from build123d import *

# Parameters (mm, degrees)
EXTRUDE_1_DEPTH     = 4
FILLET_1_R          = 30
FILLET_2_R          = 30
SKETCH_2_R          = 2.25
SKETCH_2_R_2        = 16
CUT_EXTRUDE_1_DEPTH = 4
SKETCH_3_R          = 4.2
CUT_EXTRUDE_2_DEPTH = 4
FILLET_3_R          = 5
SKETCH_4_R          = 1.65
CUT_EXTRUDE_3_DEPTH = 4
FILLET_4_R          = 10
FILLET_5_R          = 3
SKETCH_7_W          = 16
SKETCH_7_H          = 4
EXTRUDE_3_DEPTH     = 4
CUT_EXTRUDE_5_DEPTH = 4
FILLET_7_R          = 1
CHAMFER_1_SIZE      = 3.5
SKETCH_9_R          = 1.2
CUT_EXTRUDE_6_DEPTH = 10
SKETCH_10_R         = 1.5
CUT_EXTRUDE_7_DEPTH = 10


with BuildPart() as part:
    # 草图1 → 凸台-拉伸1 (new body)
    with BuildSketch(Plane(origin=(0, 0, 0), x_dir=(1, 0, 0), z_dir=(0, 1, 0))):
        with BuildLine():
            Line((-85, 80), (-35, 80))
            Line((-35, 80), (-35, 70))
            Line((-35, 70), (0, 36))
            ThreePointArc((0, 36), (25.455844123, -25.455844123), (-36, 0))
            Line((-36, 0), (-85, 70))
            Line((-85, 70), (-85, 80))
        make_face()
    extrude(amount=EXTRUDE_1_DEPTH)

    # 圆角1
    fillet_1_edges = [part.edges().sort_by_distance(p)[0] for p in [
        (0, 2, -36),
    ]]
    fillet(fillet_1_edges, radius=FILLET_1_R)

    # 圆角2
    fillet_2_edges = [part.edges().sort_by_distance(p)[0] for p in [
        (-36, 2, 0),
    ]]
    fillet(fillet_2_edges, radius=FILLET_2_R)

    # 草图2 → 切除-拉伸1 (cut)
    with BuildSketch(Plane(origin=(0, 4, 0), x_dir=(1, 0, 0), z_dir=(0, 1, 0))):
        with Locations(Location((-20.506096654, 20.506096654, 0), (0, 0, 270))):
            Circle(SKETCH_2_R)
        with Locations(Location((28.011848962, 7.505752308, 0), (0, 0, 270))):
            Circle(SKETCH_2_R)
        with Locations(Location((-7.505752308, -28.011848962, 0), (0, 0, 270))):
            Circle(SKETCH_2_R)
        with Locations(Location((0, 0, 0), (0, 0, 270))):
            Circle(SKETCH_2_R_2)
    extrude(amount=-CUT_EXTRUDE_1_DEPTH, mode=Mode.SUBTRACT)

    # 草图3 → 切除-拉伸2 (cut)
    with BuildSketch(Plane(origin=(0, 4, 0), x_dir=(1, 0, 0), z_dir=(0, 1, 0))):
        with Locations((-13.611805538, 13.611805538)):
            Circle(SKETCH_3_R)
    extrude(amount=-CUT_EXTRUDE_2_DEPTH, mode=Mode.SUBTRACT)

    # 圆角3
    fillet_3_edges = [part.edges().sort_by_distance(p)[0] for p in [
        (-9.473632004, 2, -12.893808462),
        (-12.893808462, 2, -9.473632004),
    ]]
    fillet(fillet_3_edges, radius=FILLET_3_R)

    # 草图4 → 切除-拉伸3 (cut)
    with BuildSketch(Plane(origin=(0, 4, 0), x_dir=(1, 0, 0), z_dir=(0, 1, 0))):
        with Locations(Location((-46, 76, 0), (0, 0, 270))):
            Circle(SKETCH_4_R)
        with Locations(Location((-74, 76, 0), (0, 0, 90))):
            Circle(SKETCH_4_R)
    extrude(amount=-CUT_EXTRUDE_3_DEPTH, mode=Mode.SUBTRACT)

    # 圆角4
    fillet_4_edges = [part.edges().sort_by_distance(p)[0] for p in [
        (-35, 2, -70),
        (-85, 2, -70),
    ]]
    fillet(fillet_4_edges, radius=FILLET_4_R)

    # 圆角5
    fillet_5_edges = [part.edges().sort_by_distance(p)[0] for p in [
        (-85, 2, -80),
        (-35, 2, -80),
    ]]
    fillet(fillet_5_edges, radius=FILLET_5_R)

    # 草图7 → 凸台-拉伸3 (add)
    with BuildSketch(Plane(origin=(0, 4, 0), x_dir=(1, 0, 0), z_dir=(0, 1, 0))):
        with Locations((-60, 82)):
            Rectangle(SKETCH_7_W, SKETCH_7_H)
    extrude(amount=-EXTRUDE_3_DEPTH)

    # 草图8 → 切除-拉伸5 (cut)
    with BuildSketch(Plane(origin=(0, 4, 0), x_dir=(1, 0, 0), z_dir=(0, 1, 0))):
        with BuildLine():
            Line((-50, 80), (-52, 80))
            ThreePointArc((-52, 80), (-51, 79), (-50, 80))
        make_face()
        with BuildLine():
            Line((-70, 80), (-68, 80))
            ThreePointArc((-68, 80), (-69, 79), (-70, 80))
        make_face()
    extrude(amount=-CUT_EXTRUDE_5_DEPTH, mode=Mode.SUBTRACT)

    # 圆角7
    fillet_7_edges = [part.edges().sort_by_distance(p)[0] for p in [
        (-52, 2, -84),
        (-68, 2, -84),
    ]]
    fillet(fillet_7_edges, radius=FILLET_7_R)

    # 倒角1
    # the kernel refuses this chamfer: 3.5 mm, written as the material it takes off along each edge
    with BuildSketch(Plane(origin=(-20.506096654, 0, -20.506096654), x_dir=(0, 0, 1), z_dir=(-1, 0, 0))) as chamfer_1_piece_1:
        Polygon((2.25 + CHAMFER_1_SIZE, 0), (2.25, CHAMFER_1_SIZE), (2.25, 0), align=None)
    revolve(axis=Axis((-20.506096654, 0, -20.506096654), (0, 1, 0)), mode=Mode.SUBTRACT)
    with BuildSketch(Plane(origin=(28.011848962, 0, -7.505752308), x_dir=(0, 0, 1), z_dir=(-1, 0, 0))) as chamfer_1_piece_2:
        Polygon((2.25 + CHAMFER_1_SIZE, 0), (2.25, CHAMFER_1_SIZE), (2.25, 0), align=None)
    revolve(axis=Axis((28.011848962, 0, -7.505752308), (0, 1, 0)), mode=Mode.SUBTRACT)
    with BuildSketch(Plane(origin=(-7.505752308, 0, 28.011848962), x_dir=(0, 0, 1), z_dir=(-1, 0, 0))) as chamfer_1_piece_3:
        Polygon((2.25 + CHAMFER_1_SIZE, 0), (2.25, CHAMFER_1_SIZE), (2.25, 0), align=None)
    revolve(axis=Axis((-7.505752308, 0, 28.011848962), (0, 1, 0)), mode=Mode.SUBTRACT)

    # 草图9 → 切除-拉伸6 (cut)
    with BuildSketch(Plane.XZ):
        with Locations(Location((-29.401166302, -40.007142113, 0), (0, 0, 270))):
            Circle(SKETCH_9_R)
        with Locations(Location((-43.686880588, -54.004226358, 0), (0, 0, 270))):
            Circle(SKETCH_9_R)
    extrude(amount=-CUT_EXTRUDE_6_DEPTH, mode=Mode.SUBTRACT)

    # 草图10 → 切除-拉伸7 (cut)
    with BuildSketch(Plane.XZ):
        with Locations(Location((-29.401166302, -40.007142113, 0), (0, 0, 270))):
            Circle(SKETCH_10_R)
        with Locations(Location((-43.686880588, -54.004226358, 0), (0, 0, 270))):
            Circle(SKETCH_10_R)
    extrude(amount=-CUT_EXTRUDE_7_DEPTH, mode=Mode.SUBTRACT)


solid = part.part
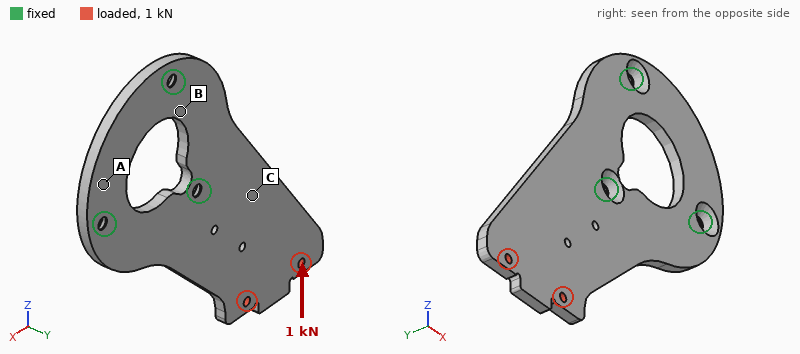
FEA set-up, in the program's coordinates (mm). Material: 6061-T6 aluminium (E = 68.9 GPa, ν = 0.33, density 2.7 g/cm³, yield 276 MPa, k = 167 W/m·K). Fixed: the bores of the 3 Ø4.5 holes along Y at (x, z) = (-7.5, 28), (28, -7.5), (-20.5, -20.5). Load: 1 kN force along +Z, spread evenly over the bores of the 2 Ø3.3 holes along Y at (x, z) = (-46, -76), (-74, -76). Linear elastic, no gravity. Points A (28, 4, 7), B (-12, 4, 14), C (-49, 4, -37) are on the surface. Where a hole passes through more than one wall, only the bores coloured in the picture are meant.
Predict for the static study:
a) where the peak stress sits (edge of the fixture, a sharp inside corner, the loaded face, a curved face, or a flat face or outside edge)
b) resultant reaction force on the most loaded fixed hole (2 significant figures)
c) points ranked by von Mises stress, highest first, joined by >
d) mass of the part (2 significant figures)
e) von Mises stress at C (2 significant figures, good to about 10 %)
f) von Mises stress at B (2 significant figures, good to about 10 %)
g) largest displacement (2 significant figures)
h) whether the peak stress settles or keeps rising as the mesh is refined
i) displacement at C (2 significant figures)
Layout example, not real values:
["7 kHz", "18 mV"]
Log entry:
["edge of the fixture", "890 N", "B > C > A", "67 g", "13 MPa", "24 MPa", "0.11 mm", "keeps rising", "0.035 mm"]
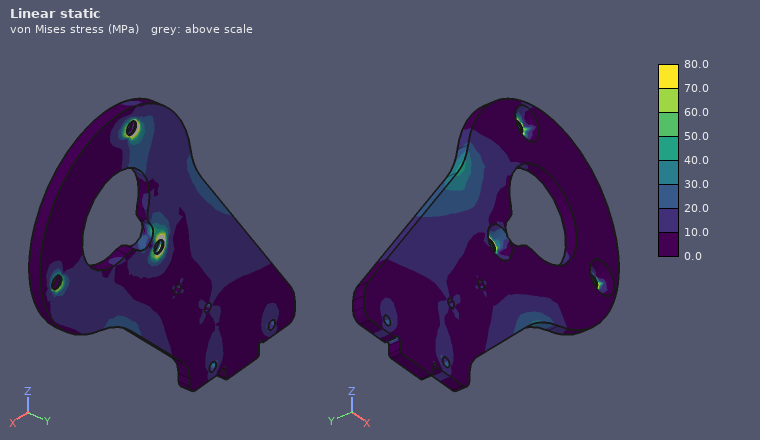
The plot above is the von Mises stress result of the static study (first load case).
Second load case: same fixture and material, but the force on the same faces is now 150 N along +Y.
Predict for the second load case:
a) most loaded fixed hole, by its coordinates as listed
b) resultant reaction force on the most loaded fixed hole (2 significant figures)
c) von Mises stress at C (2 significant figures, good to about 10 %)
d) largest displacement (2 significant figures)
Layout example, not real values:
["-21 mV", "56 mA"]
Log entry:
["(-20.5, -20.5)", "1.1 kN", "46 MPa", "1.7 mm"]
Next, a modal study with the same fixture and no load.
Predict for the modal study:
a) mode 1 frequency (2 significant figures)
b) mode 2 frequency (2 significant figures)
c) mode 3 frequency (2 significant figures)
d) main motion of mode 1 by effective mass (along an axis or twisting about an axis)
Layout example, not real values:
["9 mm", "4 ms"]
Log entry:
["480 Hz", "1400 Hz", "2600 Hz", "along Y"]
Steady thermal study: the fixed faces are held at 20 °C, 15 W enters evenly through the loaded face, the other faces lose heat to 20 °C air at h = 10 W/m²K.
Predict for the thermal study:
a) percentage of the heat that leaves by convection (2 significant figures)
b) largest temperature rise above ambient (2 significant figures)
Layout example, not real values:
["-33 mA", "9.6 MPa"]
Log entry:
["14 %", "44 K"]
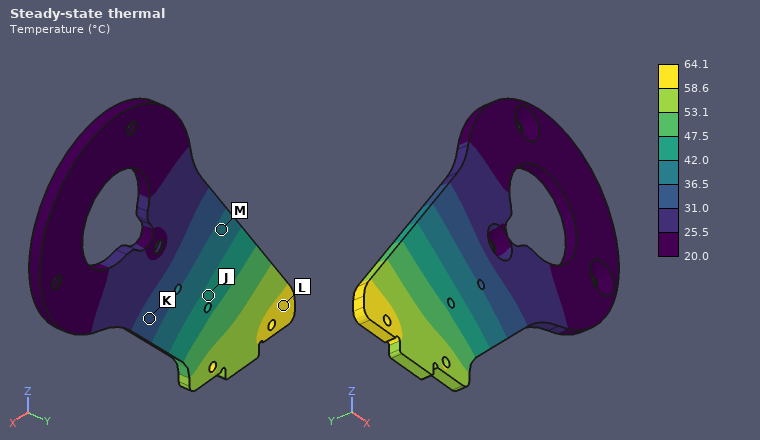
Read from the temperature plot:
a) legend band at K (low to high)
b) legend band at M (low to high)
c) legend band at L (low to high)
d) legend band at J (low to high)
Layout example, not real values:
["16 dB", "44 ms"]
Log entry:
["31.0 to 36.5 °C", "36.5 to 42.0 °C", "58.6 to 64.1 °C", "42.0 to 47.5 °C"]
